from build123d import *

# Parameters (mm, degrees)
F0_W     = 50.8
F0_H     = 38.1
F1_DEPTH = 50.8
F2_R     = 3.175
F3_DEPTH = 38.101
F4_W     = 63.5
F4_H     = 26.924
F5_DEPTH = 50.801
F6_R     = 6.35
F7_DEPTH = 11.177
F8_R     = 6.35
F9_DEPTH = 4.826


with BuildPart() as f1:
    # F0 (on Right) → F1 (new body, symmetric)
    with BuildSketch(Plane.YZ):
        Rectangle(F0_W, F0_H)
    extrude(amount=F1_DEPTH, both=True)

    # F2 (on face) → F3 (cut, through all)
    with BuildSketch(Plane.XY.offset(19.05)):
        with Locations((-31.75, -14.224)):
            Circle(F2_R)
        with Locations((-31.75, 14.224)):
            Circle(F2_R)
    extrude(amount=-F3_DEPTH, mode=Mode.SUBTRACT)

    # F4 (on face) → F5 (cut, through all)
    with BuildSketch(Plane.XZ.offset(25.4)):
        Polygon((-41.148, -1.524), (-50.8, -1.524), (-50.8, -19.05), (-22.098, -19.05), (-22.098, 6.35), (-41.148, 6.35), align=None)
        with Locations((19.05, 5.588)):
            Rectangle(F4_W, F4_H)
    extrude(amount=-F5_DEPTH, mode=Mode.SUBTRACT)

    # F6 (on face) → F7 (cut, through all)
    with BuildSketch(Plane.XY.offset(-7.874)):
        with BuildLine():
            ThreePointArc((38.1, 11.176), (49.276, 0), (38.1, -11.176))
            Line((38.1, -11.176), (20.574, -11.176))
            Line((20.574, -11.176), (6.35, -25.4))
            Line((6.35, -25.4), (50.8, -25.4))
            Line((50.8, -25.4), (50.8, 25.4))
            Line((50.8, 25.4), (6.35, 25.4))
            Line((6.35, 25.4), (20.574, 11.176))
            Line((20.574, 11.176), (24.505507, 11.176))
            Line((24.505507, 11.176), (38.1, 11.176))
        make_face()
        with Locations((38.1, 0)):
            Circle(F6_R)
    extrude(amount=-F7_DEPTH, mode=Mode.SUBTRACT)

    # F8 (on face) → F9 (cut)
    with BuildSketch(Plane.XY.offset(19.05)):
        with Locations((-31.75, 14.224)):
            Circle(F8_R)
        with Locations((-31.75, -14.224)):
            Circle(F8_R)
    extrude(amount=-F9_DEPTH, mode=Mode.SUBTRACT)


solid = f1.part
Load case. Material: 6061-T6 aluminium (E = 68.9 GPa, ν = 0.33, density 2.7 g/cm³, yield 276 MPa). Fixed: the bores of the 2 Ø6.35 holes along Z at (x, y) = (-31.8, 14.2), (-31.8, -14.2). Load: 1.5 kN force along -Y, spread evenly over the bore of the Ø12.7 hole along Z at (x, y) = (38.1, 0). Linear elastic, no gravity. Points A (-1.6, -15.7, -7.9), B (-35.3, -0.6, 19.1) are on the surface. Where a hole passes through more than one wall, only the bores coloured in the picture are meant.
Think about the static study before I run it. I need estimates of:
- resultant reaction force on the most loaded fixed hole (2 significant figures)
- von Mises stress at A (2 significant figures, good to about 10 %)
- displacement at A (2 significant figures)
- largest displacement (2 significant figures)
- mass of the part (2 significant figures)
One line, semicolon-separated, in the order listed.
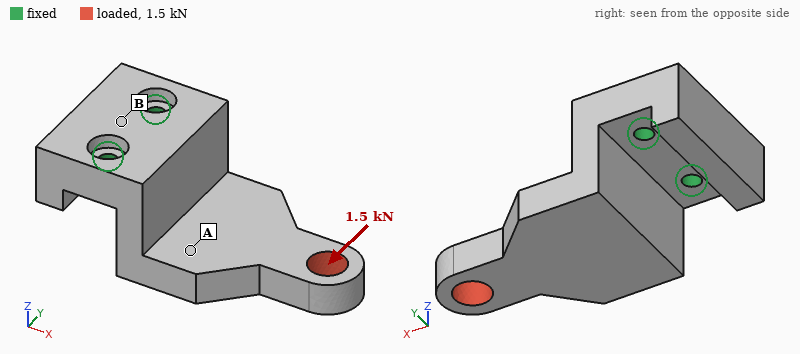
3.6 kN; 27 MPa; 0.063 mm; 0.22 mm; 160 g
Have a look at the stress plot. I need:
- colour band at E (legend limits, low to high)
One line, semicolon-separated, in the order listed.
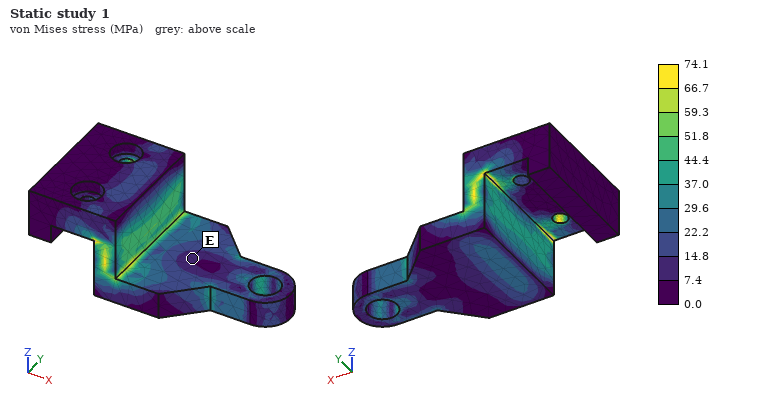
7.4 to 14.8 MPa
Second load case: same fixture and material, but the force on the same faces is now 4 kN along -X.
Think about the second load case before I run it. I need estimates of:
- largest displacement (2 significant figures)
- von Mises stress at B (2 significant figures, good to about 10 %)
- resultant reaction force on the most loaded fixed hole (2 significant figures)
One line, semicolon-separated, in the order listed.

0.65 mm; 24 MPa; 2.1 kN
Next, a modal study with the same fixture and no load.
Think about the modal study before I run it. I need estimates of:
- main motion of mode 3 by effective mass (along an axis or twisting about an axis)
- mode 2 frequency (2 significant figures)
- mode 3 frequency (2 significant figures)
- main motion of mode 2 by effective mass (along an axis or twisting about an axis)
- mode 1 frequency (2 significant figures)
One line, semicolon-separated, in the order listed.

along X; 3300 Hz; 5000 Hz; along Y; 1400 Hz
